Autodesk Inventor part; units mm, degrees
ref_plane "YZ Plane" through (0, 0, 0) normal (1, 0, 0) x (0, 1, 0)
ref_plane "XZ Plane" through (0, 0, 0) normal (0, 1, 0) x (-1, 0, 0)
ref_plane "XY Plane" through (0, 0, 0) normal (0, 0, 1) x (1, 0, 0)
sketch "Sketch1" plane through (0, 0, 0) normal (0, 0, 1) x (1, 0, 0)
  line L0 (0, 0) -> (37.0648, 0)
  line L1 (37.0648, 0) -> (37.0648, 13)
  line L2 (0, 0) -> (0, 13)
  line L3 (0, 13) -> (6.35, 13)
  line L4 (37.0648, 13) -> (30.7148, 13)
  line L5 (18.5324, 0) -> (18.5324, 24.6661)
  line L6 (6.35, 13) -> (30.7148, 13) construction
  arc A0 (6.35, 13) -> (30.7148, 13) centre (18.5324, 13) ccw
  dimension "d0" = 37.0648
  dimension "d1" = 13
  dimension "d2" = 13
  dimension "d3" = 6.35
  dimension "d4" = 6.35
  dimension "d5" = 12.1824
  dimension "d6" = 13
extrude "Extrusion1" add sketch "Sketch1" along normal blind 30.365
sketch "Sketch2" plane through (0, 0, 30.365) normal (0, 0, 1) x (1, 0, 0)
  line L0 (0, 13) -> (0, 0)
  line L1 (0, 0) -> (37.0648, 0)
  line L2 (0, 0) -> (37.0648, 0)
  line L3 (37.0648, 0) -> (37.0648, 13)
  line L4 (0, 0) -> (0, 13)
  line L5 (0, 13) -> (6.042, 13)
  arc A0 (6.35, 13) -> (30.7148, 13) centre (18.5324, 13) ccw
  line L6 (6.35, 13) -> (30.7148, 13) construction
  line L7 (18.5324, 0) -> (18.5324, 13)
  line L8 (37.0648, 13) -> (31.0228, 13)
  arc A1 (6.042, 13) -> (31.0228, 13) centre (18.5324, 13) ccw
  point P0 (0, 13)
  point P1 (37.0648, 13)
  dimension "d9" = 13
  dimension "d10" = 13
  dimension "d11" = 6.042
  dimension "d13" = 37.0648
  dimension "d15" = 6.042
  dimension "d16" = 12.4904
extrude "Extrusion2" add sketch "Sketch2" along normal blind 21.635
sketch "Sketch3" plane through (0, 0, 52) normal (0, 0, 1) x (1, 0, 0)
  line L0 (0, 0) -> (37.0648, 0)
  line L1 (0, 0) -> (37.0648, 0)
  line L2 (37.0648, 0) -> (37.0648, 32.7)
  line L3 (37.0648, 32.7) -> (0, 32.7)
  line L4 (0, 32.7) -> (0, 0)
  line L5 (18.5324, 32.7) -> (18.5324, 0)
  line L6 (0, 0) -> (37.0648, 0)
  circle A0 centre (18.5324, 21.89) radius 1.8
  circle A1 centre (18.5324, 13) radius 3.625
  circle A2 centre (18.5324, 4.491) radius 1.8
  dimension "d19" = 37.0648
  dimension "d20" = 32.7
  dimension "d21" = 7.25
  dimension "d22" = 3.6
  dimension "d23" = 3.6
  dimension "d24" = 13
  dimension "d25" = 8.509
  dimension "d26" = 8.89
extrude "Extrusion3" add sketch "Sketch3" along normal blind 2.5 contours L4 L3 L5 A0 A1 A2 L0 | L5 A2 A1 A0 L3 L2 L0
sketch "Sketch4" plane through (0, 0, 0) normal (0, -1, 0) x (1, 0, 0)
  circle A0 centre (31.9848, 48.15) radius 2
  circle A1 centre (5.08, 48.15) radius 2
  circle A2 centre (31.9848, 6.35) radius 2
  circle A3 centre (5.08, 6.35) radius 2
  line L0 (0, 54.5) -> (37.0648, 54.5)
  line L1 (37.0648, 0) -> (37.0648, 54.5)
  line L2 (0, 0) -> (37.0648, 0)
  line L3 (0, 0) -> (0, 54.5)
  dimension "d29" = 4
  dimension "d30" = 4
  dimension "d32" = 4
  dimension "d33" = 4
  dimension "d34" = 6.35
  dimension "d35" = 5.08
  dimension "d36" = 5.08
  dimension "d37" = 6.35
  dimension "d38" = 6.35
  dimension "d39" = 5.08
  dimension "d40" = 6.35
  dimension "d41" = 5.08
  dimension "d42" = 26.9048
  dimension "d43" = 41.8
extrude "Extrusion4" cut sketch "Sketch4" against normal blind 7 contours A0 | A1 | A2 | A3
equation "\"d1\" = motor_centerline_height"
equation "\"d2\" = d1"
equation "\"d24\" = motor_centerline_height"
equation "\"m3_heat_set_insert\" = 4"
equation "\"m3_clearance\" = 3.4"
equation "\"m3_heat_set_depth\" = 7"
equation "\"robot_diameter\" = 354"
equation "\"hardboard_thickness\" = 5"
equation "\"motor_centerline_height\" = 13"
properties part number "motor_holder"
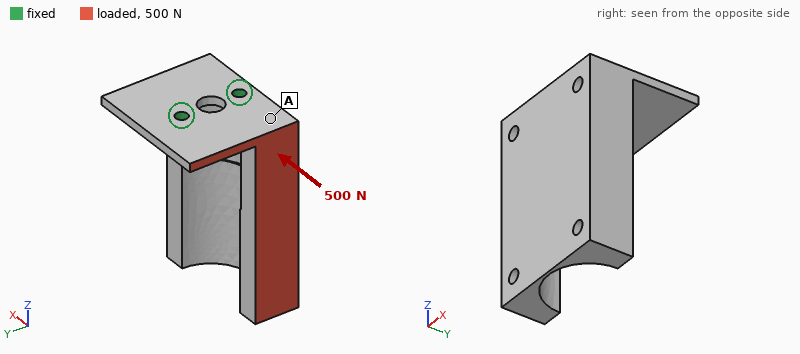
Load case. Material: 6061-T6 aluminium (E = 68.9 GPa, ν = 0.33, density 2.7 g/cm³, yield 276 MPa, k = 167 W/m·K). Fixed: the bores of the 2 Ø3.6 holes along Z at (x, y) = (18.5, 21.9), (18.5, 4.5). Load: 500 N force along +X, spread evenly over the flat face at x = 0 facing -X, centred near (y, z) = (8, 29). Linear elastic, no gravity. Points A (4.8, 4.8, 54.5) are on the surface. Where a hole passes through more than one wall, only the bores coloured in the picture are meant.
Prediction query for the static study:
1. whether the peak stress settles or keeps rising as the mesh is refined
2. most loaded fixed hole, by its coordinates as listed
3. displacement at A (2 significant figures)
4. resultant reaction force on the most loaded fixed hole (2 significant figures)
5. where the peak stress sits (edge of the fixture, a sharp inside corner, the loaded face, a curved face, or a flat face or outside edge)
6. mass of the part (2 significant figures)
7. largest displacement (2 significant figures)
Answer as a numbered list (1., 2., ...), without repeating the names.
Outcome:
1. keeps rising
2. (18.5, 4.5)
3. 0.13 mm
4. 370 N
5. edge of the fixture
6. 41 g
7. 0.58 mm
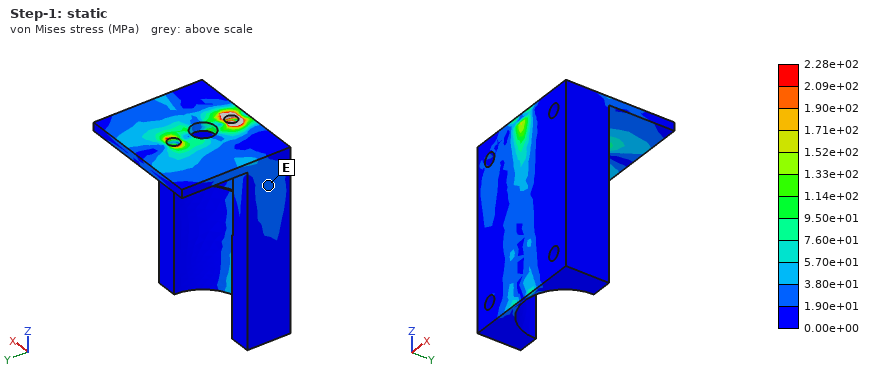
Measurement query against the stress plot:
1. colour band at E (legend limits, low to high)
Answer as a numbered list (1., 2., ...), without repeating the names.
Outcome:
1. 1.90e+01 to 3.80e+01 MPa
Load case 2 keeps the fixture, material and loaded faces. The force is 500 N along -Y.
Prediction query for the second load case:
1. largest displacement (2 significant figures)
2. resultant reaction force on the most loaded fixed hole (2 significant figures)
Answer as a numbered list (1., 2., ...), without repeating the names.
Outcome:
1. 0.53 mm
2. 770 N
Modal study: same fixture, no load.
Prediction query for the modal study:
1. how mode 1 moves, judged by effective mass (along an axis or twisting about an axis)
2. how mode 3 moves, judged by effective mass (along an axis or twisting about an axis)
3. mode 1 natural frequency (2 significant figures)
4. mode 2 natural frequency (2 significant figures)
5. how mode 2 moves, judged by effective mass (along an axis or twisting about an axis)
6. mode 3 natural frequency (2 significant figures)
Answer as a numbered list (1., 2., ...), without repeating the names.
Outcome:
1. along X
2. twisting about Z
3. 900 Hz
4. 1100 Hz
5. along Y
6. 2900 Hz
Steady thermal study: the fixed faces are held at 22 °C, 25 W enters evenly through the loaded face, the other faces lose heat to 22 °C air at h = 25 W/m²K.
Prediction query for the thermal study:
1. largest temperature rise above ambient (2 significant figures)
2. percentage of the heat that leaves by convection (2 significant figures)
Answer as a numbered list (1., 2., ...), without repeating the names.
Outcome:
1. 35 K
2. 14 %
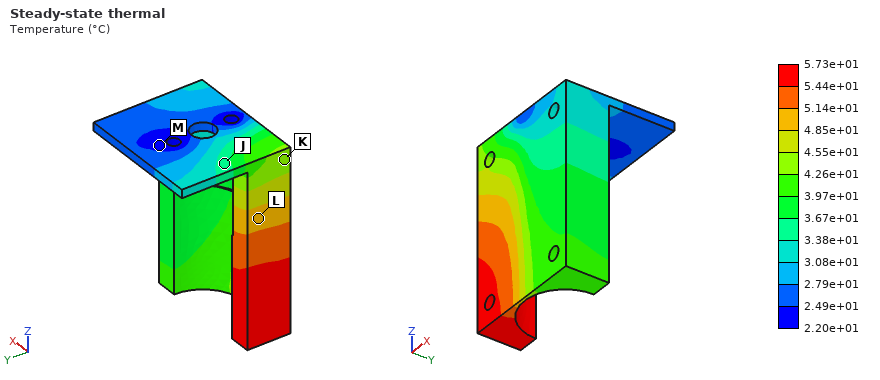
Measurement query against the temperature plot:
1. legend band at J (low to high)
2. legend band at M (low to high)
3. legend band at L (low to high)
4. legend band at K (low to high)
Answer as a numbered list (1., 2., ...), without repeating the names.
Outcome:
1. 3.38e+01 to 3.67e+01 °C
2. 2.20e+01 to 2.49e+01 °C
3. 4.85e+01 to 5.14e+01 °C
4. 4.26e+01 to 4.55e+01 °C
